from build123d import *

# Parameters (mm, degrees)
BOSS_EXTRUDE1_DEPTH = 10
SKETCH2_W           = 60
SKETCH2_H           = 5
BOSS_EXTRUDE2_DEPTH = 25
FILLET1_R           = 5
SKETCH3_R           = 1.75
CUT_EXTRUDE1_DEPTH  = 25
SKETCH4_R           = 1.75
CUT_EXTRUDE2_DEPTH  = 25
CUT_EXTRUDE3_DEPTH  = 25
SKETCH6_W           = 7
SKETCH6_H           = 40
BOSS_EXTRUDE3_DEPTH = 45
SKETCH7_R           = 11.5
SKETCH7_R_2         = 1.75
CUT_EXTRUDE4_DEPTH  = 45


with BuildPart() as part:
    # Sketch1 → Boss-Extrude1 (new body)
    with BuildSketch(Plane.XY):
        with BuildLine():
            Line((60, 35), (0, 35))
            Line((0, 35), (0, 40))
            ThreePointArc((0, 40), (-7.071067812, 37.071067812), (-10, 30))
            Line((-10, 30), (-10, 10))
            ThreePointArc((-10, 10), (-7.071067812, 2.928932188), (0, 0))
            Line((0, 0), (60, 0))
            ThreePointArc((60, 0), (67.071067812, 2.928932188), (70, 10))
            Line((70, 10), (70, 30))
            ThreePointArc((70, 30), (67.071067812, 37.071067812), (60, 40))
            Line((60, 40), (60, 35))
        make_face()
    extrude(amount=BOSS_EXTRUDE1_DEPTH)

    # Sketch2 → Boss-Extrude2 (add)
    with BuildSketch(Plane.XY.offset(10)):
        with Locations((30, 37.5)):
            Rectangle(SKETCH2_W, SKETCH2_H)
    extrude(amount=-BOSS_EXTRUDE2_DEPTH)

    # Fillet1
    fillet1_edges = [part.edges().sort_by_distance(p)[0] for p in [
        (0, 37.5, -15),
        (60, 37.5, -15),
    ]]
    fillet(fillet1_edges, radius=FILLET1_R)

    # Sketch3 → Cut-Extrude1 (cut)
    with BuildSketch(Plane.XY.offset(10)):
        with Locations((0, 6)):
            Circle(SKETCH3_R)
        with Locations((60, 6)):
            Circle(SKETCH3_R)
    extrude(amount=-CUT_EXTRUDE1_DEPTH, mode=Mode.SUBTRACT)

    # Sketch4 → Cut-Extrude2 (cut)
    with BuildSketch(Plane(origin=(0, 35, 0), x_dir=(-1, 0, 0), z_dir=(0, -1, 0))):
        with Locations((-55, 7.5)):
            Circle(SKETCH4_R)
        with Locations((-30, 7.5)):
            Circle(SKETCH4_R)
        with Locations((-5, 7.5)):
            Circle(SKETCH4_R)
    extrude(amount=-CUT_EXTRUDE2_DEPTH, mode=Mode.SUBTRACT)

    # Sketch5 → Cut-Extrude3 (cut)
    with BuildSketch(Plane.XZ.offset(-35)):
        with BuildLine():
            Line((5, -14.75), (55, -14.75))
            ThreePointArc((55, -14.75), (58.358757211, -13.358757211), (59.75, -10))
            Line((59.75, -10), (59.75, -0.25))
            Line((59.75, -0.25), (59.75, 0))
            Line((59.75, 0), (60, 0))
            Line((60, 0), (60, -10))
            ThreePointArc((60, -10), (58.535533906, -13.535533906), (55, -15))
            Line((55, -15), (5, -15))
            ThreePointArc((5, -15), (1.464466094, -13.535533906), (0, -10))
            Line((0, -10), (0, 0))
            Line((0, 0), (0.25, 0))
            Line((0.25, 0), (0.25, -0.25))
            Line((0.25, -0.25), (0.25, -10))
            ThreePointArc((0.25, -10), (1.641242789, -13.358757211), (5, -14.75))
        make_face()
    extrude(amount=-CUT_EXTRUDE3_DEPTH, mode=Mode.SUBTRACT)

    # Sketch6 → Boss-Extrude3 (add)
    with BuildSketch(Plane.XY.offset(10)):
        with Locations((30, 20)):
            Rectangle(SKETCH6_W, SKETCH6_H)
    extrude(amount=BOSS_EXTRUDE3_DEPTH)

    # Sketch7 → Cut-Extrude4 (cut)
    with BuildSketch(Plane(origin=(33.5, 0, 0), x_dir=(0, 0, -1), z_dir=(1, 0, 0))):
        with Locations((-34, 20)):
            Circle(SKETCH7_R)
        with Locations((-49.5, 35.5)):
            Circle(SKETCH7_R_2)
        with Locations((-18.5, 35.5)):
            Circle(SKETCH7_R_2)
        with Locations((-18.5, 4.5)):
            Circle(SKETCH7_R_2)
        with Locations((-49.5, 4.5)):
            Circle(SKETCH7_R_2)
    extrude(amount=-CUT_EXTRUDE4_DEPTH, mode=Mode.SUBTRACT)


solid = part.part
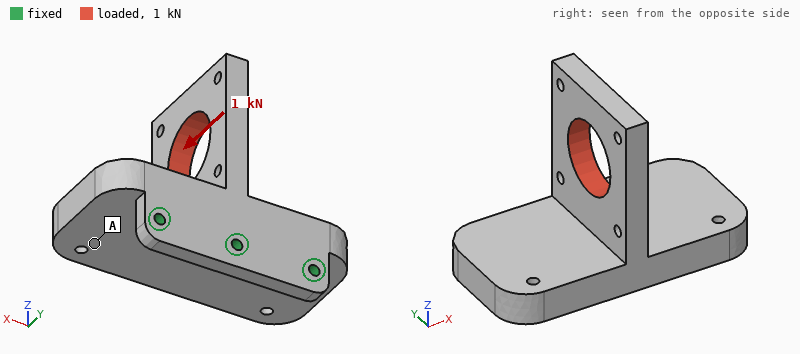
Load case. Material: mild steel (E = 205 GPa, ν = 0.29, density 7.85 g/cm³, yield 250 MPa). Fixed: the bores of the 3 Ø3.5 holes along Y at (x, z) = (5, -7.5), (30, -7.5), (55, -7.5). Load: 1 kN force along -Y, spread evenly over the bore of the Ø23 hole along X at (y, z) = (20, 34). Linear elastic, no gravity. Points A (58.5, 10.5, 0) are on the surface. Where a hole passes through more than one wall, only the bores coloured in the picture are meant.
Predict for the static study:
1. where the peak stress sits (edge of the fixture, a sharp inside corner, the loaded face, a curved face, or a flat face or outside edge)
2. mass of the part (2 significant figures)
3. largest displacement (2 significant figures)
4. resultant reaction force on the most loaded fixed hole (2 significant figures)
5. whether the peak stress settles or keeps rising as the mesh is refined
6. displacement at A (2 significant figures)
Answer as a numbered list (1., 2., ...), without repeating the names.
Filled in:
1. edge of the fixture
2. 350 g
3. 0.24 mm
4. 400 N
5. keeps rising
6. 0.088 mm
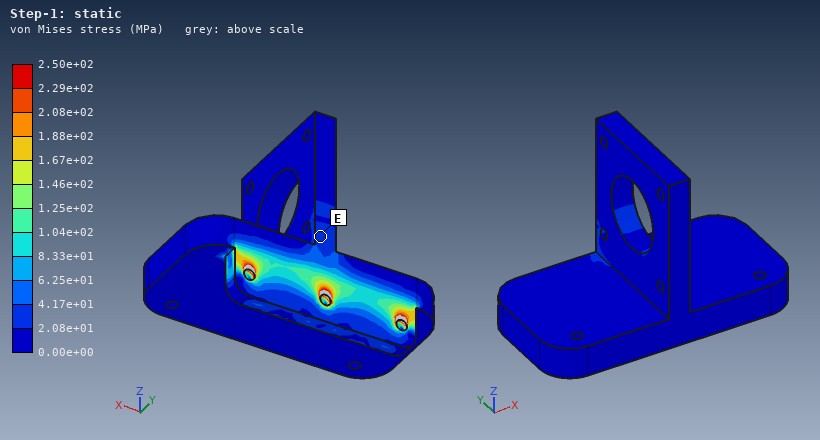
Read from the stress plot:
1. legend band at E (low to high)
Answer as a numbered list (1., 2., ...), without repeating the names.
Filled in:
1. 2.08e+01 to 4.17e+01 MPa
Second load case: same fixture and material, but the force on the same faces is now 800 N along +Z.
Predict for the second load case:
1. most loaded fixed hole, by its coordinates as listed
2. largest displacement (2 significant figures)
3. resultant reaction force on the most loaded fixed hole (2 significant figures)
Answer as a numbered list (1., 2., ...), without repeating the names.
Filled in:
1. (30, -7.5)
2. 87 µm
3. 520 N
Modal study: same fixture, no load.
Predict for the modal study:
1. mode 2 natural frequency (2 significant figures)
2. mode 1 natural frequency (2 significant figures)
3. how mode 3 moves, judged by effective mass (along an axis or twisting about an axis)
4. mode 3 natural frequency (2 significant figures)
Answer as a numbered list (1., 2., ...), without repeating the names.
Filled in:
1. 2300 Hz
2. 1000 Hz
3. along X
4. 4000 Hz
